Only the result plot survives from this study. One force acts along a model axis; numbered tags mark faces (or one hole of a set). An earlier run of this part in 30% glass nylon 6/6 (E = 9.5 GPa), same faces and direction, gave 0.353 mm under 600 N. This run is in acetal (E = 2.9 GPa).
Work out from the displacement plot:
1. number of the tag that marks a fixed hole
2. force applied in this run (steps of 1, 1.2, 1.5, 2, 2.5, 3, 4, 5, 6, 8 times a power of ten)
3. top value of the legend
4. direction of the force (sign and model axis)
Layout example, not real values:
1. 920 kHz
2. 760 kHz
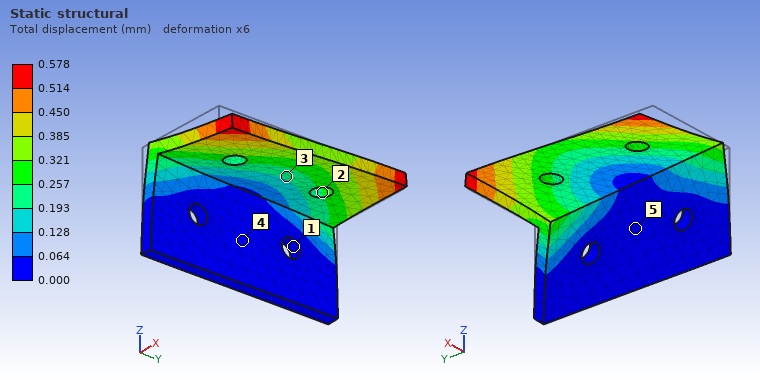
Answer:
1. 1
2. 300 N
3. 0.578 mm
4. +Y
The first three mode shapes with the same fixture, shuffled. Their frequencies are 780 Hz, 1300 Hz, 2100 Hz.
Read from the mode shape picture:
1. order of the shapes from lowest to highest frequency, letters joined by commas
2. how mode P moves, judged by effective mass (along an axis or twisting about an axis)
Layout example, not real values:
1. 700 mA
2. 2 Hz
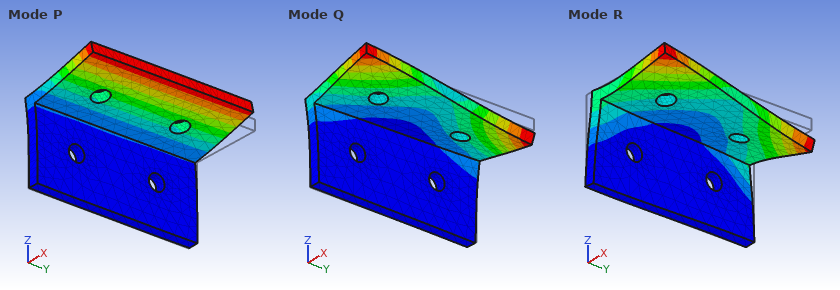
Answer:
1. P, Q, R
2. along Z
